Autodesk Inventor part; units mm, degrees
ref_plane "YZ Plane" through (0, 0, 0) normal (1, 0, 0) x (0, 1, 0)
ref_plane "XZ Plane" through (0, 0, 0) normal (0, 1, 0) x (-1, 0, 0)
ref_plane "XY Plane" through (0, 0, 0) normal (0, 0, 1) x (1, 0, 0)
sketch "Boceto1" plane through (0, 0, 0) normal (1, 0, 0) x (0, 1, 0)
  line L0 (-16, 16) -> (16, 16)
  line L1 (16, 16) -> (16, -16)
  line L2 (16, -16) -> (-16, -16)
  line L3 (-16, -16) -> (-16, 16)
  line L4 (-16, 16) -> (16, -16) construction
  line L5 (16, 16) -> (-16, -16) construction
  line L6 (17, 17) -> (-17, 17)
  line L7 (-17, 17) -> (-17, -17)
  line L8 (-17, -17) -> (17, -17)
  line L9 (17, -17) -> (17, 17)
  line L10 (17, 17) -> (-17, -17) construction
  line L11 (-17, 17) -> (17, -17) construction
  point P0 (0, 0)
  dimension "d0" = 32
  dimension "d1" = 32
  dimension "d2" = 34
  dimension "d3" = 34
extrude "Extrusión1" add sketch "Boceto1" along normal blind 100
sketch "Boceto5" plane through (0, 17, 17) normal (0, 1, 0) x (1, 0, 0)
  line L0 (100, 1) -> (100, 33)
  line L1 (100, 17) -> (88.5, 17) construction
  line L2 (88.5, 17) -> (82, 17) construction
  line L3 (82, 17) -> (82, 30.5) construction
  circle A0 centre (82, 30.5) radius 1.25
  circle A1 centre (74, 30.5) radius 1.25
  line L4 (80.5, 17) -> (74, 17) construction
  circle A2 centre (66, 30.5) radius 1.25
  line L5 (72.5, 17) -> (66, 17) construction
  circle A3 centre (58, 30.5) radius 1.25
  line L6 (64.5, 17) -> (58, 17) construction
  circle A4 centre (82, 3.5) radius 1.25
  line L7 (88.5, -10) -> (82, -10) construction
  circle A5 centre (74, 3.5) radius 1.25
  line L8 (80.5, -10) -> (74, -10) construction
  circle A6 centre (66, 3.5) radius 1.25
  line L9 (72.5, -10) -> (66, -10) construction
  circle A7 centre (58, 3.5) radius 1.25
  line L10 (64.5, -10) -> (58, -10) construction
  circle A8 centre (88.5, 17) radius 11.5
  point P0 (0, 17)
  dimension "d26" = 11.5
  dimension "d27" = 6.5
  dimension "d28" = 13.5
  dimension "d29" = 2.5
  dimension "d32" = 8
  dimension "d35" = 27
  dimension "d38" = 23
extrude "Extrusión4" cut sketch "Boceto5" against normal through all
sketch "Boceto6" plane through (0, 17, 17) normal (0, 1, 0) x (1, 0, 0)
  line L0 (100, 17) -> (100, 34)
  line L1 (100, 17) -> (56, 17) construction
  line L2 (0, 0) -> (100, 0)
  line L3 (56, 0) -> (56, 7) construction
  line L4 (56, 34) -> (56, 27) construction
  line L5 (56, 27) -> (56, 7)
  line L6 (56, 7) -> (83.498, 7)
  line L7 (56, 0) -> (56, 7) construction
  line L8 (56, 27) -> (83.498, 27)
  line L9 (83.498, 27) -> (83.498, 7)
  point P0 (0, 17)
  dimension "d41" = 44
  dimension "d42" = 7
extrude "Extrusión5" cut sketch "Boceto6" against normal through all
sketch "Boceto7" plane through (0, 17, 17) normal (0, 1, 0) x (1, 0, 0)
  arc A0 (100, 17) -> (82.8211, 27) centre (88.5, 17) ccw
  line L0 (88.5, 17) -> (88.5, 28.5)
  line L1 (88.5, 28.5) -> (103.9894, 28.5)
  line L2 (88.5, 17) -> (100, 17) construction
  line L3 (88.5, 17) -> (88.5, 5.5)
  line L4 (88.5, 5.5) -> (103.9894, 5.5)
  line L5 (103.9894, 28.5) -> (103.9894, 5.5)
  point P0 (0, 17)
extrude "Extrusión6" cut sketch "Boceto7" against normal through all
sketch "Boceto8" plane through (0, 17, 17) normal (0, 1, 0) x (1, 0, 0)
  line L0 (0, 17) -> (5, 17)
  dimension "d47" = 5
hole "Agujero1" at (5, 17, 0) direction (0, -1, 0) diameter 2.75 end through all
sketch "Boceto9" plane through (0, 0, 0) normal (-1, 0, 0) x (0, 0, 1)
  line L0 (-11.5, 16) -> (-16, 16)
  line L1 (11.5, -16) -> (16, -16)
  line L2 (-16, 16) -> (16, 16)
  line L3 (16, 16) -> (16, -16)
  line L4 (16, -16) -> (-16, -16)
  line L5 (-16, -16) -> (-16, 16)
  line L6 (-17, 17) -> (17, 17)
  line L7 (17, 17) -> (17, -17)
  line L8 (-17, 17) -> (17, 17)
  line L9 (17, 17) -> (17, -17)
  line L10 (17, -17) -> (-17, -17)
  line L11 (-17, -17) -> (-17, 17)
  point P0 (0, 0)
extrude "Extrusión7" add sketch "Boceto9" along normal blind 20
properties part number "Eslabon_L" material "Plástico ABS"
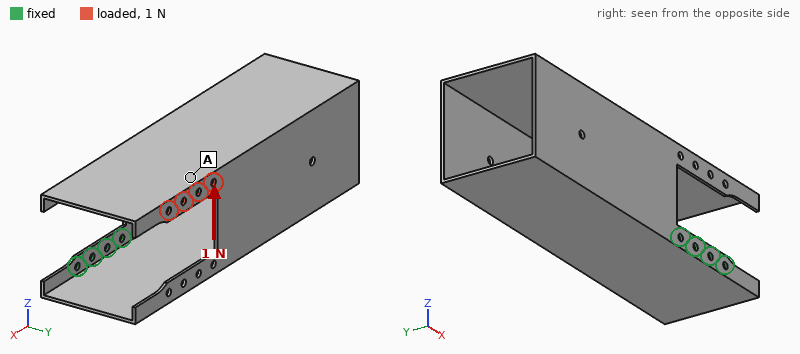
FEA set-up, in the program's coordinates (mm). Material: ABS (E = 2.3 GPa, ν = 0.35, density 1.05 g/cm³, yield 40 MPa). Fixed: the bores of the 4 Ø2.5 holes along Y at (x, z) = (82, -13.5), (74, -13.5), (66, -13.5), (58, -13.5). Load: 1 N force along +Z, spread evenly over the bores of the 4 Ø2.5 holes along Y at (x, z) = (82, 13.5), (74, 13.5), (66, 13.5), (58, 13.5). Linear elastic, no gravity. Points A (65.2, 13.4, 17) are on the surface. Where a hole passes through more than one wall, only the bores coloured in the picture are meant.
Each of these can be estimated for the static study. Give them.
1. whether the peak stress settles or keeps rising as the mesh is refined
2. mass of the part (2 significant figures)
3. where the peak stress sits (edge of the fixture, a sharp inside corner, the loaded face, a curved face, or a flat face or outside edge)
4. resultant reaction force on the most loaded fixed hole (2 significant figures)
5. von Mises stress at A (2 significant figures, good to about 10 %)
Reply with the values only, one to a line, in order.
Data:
keeps rising
15 g
edge of the fixture
1.2 N
0.38 MPa
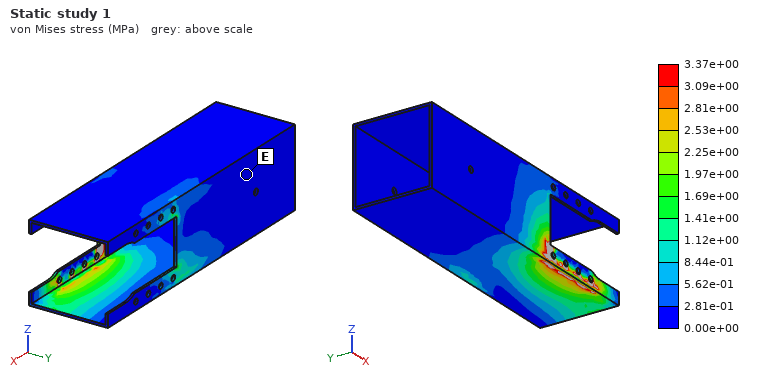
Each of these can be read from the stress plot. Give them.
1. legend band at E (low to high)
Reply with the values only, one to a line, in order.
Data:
0.00e+00 to 2.81e-01 MPa
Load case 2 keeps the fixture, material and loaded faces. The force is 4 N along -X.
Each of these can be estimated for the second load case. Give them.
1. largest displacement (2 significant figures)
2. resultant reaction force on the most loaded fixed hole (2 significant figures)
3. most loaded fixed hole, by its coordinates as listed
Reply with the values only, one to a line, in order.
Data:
1.3 mm
11 N
(58, -13.5)
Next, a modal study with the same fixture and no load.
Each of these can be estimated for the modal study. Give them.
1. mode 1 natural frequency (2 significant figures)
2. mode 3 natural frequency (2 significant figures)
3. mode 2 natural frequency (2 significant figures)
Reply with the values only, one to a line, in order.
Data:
45 Hz
160 Hz
110 Hz
